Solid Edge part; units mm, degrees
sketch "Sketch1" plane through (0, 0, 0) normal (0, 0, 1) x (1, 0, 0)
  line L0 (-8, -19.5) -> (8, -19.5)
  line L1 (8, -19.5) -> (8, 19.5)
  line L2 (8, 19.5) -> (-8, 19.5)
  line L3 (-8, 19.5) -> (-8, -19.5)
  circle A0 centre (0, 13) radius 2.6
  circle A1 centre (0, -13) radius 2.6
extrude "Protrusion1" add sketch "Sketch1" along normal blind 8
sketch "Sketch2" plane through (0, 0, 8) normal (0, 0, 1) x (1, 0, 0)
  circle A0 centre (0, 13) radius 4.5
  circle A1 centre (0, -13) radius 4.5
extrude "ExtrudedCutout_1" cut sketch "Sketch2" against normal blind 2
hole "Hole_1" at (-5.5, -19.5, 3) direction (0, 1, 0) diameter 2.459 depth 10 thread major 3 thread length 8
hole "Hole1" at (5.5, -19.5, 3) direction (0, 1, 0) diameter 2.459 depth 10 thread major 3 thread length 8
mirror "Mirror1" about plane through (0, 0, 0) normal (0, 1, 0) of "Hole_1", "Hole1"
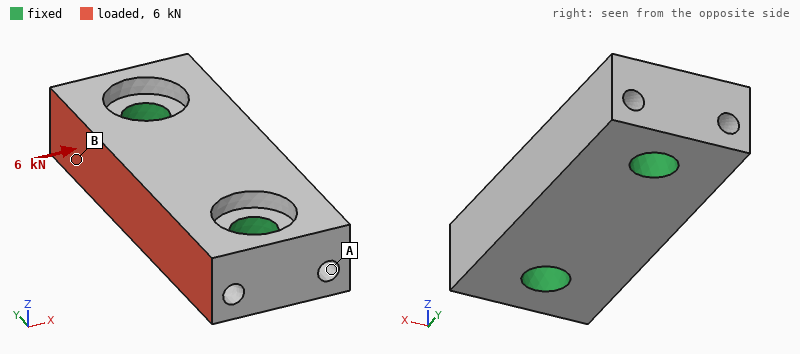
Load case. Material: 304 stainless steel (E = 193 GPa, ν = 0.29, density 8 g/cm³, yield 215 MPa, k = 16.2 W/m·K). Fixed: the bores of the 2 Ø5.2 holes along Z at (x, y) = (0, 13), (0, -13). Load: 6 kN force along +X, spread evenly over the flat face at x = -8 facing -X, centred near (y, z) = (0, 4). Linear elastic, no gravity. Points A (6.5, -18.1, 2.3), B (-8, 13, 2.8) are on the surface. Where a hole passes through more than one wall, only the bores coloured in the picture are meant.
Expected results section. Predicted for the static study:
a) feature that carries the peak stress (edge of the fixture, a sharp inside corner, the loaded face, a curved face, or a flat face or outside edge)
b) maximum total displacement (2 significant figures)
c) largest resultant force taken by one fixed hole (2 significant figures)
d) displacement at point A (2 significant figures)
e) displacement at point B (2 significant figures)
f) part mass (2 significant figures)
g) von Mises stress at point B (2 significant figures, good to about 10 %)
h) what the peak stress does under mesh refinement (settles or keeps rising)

edge of the fixture
3.6 µm
3.0 kN
0.54 µm
1.7 µm
34 g
24 MPa
keeps rising
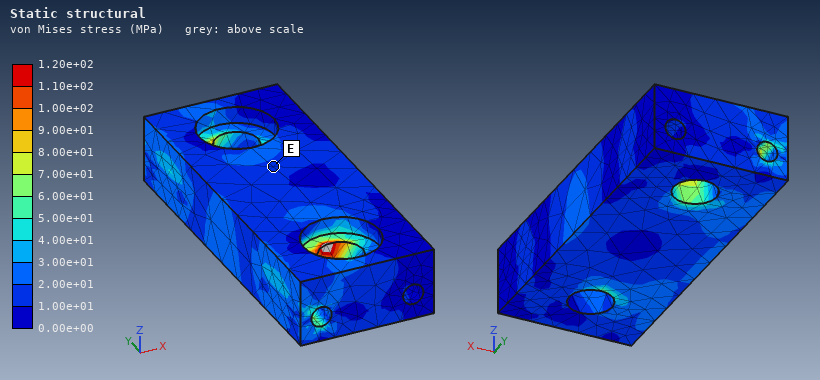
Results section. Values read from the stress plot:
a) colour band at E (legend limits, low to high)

1.00e+01 to 2.00e+01 MPa
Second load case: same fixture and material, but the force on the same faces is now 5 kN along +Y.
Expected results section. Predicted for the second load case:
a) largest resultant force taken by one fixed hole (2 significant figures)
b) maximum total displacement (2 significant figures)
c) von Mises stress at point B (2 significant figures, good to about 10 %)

2.8 kN
4.5 µm
35 MPa
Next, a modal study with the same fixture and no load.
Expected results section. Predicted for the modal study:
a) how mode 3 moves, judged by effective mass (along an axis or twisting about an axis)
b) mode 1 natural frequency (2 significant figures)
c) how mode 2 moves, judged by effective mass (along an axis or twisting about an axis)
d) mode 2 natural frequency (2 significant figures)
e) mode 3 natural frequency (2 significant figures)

along X
35 kHz
along Z
37 kHz
45 kHz
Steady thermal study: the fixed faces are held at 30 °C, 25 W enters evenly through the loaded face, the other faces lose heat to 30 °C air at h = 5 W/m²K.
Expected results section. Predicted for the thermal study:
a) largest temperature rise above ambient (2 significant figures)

61 K
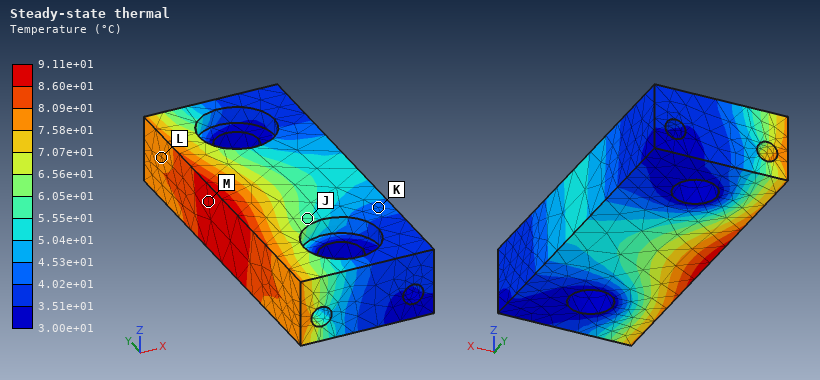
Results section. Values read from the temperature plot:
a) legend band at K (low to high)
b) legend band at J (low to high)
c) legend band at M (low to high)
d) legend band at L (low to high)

4.02e+01 to 4.53e+01 °C
5.55e+01 to 6.05e+01 °C
8.60e+01 to 9.11e+01 °C
7.58e+01 to 8.09e+01 °C
